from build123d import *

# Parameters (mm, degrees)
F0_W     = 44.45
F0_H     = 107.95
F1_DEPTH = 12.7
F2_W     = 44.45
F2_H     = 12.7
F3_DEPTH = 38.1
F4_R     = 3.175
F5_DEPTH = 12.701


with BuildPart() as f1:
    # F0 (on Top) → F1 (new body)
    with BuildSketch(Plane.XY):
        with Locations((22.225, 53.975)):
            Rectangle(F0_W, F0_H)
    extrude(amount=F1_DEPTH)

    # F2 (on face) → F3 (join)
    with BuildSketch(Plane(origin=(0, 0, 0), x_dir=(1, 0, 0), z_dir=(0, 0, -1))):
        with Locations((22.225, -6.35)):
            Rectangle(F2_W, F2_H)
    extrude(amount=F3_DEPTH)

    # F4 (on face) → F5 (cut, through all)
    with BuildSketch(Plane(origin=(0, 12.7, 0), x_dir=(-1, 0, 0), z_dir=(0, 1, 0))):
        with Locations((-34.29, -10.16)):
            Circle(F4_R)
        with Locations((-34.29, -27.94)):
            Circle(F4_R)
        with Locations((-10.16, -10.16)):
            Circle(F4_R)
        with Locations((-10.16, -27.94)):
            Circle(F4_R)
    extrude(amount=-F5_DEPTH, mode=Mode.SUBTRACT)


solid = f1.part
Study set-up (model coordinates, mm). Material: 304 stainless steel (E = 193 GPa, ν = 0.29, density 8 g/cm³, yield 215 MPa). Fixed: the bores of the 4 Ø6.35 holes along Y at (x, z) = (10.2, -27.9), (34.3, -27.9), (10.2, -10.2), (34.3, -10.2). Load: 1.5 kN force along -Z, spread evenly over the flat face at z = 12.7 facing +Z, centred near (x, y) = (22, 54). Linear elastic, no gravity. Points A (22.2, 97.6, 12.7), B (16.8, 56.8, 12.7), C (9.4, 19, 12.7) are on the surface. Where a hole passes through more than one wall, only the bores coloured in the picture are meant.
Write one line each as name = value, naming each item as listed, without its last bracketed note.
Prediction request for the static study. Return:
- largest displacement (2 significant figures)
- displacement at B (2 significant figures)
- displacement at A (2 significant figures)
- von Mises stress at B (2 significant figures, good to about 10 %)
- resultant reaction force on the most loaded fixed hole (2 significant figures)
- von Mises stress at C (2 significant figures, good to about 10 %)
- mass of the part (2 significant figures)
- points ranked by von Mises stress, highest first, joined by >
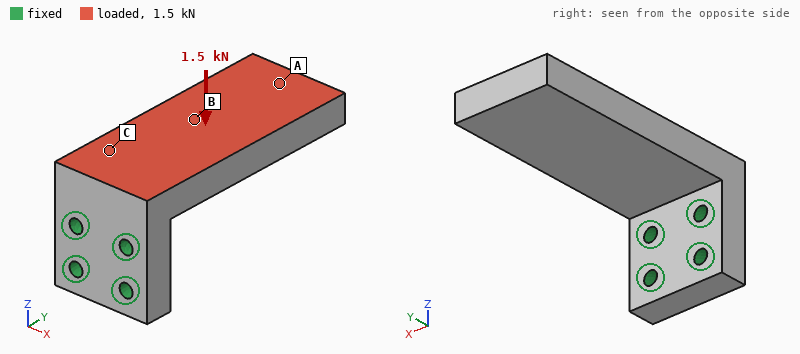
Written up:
largest displacement = 0.19 mm
displacement at B = 0.076 mm
displacement at A = 0.16 mm
von Mises stress at B = 15 MPa
resultant reaction force on the most loaded fixed hole = 830 N
von Mises stress at C = 45 MPa
mass of the part = 650 g
points ranked by von Mises stress, highest first, joined by > = C > B > A
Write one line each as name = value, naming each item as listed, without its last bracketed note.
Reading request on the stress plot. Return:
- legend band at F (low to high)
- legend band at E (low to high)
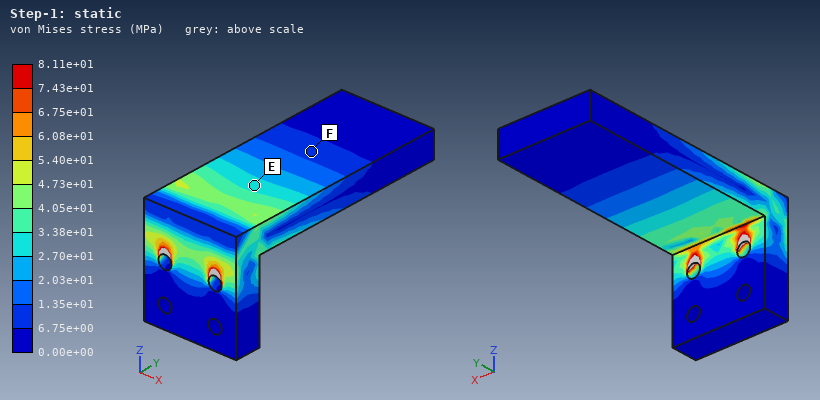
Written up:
legend band at F = 6.75e+00 to 1.35e+01 MPa
legend band at E = 2.70e+01 to 3.38e+01 MPa
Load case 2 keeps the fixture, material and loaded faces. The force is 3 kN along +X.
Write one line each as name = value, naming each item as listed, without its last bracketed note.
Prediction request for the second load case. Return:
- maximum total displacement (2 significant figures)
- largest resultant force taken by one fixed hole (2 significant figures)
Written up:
maximum total displacement = 68 µm
largest resultant force taken by one fixed hole = 5.0 kN
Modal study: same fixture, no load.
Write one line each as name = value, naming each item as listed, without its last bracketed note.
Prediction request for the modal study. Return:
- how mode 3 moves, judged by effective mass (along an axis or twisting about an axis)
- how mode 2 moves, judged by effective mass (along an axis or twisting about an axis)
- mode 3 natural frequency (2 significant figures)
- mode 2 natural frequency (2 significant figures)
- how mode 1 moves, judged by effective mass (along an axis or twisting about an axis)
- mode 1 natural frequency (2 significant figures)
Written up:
how mode 3 moves, judged by effective mass = twisting about Y
how mode 2 moves, judged by effective mass = along X
mode 3 natural frequency = 4000 Hz
mode 2 natural frequency = 1800 Hz
how mode 1 moves, judged by effective mass = along Z
mode 1 natural frequency = 800 Hz
